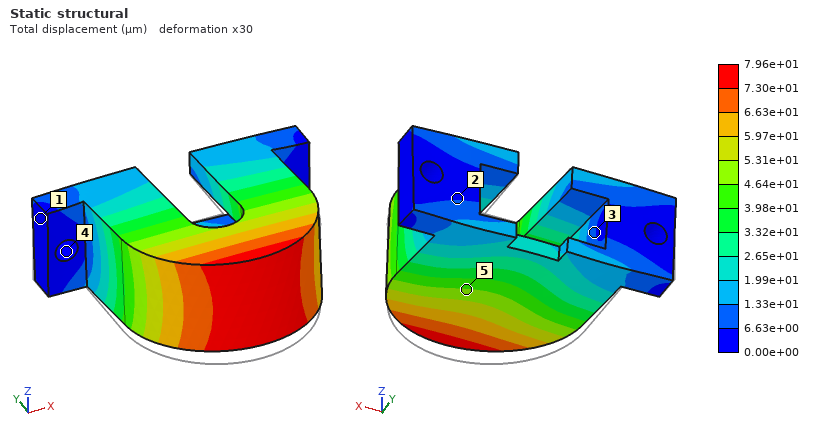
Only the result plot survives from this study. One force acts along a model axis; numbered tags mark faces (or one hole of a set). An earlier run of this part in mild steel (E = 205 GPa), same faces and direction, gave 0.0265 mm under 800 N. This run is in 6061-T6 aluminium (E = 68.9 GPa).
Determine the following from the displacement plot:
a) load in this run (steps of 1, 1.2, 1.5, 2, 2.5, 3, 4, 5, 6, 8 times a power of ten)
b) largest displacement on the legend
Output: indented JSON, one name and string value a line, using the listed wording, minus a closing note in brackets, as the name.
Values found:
{
  "load in this run": "800 N",
  "largest displacement on the legend": "7.96e+01 µm"
}
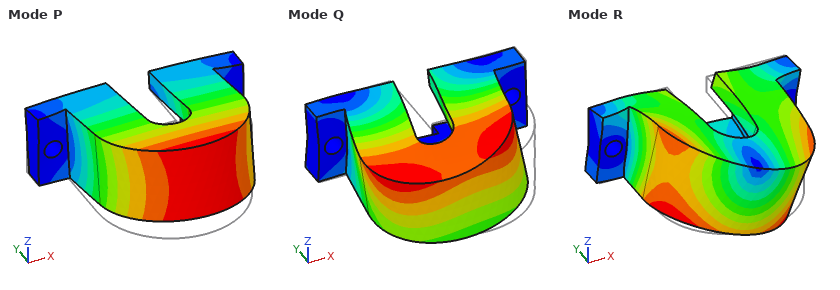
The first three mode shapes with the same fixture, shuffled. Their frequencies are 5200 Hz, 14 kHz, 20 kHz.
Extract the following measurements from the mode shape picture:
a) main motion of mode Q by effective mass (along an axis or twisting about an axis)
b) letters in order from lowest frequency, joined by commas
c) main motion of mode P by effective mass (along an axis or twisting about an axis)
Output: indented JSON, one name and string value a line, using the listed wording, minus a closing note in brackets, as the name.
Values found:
{
  "main motion of mode Q by effective mass": "along X",
  "letters in order from lowest frequency, joined by commas": "P, Q, R",
  "main motion of mode P by effective mass": "along Z"
}
